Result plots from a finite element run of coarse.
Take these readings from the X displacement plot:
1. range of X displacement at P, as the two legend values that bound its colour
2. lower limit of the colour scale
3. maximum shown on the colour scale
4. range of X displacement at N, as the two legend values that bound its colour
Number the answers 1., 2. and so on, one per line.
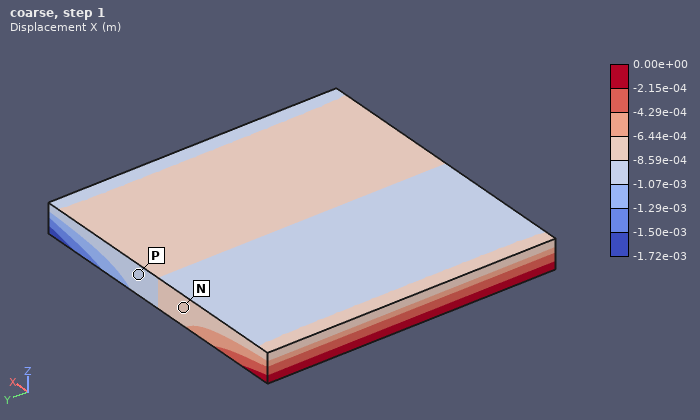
1. -1.07e-03 to -8.59e-04 m
2. -1.72e-03 m
3. 0.00e+00 m
4. -8.59e-04 to -6.44e-04 m
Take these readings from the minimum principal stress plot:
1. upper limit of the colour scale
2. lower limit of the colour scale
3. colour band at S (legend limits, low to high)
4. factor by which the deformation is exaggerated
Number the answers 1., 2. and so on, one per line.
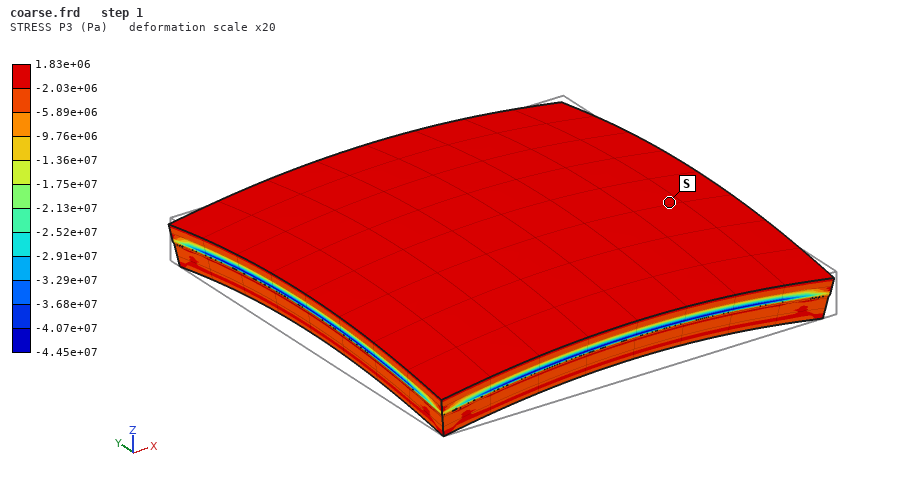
1. 1.83e+06 Pa
2. -4.45e+07 Pa
3. -2.03e+06 to 1.83e+06 Pa
4. 20
